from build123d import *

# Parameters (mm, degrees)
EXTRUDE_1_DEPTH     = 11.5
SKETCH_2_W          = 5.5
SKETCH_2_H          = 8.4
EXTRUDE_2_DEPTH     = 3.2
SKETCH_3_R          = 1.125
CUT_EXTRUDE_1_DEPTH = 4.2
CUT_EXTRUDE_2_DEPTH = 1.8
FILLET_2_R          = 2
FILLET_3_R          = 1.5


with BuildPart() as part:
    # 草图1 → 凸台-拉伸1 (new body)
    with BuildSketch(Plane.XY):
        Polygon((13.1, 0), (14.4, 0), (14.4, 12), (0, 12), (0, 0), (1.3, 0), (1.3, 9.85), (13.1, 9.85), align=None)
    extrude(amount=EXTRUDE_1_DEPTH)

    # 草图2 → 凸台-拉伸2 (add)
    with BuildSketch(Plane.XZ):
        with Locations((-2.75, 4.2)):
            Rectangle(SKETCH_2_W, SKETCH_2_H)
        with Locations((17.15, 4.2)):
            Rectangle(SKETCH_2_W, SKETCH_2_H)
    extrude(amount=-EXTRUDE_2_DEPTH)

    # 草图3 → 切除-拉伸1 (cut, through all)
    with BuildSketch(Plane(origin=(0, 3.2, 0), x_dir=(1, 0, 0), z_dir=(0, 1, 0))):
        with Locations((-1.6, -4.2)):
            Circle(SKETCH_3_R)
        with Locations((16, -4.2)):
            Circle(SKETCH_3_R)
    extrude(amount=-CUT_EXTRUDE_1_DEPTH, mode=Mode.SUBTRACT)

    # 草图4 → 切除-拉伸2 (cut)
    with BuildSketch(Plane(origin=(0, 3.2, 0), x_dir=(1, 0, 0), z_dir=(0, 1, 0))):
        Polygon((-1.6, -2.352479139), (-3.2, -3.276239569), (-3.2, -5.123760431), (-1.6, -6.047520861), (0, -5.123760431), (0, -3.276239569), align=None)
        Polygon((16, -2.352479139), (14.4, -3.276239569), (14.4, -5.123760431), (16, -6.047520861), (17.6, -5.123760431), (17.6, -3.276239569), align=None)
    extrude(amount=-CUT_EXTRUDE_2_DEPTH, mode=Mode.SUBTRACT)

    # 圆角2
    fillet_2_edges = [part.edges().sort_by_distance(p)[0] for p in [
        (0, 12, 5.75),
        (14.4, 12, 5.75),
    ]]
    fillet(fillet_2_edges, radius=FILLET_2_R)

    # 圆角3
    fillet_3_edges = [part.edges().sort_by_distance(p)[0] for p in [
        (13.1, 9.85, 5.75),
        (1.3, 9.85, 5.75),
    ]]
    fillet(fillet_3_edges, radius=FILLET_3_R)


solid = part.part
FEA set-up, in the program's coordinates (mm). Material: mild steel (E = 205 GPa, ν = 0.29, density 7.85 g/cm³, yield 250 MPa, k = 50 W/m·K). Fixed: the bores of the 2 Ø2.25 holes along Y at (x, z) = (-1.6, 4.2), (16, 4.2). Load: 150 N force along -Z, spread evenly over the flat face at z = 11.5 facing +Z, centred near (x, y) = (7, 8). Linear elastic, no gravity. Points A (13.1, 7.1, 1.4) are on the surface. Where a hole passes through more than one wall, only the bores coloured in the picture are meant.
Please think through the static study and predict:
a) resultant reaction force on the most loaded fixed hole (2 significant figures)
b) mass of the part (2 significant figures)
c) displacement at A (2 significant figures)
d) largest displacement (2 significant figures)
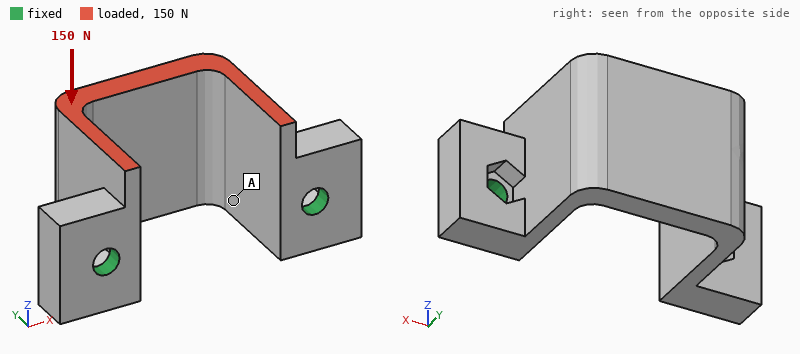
75 N
7.0 g
5.2 µm
10 µm
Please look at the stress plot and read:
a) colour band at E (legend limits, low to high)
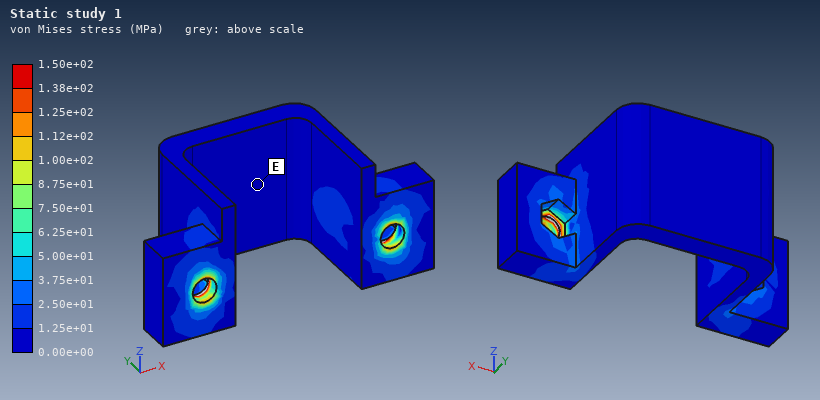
0.00e+00 to 1.25e+01 MPa
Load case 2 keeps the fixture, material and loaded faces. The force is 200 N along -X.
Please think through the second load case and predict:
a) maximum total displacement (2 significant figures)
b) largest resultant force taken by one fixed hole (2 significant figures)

15 µm
120 N
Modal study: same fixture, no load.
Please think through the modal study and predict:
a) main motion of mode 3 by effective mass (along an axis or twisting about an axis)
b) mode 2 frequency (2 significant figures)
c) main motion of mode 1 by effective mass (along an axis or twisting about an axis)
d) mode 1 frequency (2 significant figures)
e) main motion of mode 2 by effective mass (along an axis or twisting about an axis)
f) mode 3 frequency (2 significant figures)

twisting about Y
11 kHz
along Z
9500 Hz
along X
17 kHz
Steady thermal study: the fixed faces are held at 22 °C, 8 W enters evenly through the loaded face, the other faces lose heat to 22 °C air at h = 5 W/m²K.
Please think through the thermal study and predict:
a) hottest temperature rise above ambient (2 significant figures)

61 K
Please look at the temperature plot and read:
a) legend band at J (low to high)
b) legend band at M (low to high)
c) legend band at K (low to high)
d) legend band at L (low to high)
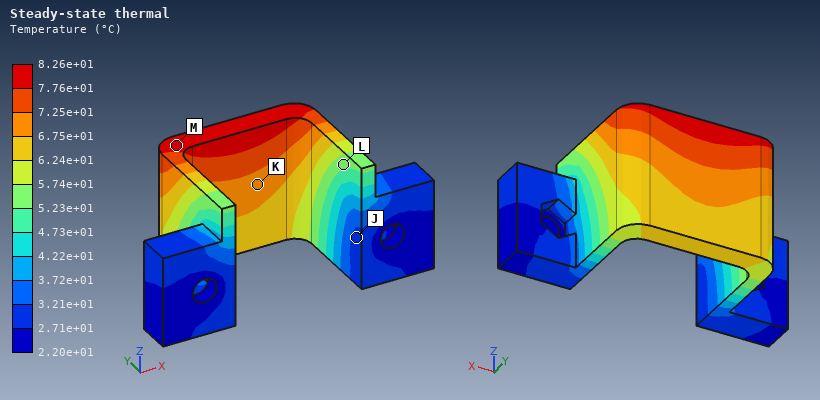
2.71e+01 to 3.21e+01 °C
7.76e+01 to 8.26e+01 °C
6.75e+01 to 7.25e+01 °C
5.23e+01 to 5.74e+01 °C
